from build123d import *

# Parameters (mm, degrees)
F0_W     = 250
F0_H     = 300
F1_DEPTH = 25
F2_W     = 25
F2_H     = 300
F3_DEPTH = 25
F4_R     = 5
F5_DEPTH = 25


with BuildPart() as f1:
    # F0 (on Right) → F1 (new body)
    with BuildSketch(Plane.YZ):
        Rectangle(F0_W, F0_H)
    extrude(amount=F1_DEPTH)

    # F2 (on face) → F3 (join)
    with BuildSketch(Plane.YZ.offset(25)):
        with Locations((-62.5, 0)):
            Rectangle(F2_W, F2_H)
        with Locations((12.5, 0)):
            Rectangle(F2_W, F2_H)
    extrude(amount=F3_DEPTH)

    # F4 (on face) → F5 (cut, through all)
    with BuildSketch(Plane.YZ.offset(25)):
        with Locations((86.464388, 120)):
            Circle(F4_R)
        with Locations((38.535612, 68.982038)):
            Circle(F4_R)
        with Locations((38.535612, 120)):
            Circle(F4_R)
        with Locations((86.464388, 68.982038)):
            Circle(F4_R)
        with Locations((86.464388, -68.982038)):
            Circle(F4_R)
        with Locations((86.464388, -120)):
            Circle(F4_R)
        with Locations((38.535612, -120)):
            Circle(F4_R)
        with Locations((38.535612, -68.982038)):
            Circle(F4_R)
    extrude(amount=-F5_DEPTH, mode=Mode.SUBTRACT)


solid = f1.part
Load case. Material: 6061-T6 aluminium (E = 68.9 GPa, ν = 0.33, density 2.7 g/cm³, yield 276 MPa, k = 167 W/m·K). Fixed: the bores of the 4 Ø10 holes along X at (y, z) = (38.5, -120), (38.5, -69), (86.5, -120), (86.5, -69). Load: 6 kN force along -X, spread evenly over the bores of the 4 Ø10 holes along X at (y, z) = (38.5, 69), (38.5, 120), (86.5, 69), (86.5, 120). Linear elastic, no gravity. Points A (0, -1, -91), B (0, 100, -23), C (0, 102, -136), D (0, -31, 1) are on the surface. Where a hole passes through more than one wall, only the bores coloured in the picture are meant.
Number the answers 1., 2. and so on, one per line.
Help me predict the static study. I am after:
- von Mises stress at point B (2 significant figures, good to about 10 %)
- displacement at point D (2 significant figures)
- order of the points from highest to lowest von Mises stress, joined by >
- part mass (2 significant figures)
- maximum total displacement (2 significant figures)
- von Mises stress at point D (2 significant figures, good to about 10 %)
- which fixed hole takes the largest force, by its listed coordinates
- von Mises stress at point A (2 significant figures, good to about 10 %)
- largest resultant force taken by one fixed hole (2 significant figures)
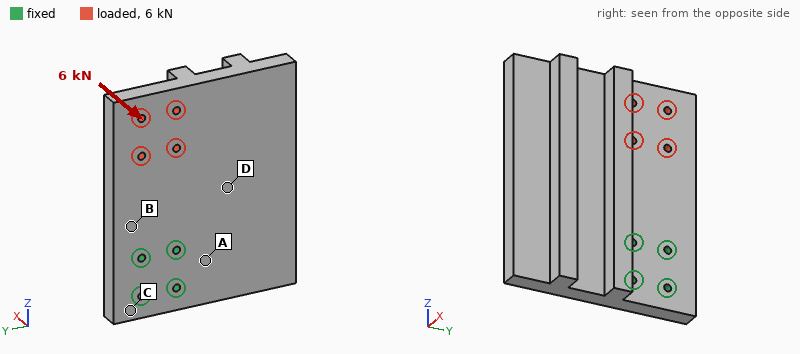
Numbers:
1. 22 MPa
2. 0.10 mm
3. B > A > D > C
4. 6.0 kg
5. 0.53 mm
6. 10 MPa
7. (38.5, -69)
8. 16 MPa
9. 12 kN
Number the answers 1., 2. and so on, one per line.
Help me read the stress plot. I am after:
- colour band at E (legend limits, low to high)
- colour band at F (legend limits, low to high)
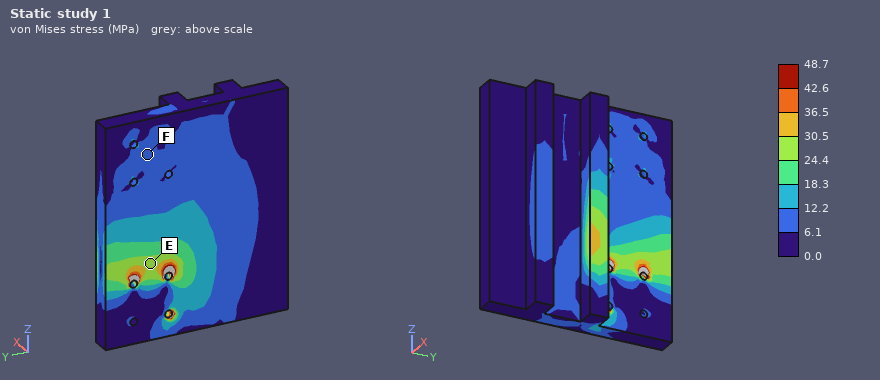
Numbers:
1. 24.4 to 30.5 MPa
2. 6.1 to 12.2 MPa
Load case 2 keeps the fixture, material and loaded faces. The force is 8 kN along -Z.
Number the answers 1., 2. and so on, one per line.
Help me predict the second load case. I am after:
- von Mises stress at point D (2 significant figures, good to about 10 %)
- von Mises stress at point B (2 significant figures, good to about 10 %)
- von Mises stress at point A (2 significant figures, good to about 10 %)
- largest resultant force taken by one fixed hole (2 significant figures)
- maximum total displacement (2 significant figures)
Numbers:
1. 0.77 MPa
2. 3.0 MPa
3. 0.95 MPa
4. 3.2 kN
5. 12 µm
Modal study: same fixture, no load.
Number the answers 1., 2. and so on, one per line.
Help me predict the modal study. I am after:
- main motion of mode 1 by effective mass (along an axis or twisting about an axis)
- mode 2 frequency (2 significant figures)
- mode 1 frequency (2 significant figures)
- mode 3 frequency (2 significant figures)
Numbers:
1. along X
2. 630 Hz
3. 370 Hz
4. 1000 Hz
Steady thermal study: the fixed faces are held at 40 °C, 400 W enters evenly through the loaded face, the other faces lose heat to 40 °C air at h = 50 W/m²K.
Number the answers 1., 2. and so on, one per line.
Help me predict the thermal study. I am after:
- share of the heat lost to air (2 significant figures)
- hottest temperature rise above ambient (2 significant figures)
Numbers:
1. 52 %
2. 61 K
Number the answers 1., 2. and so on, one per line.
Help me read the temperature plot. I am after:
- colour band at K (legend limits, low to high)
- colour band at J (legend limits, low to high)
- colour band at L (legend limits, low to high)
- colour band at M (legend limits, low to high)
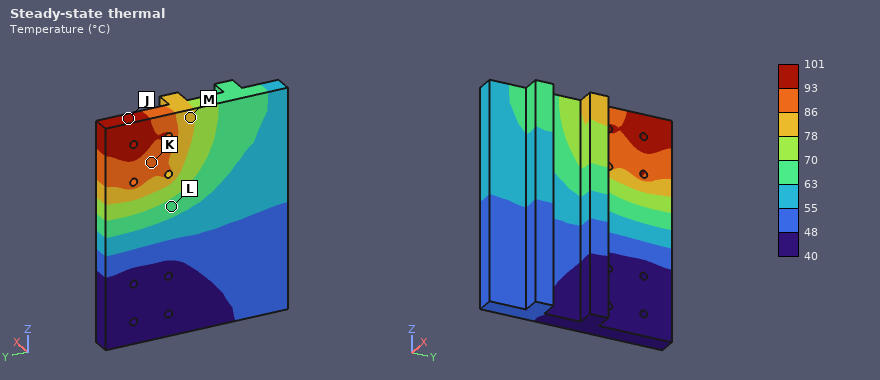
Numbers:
1. 86 to 93 °C
2. 93 to 101 °C
3. 63 to 70 °C
4. 78 to 86 °C
